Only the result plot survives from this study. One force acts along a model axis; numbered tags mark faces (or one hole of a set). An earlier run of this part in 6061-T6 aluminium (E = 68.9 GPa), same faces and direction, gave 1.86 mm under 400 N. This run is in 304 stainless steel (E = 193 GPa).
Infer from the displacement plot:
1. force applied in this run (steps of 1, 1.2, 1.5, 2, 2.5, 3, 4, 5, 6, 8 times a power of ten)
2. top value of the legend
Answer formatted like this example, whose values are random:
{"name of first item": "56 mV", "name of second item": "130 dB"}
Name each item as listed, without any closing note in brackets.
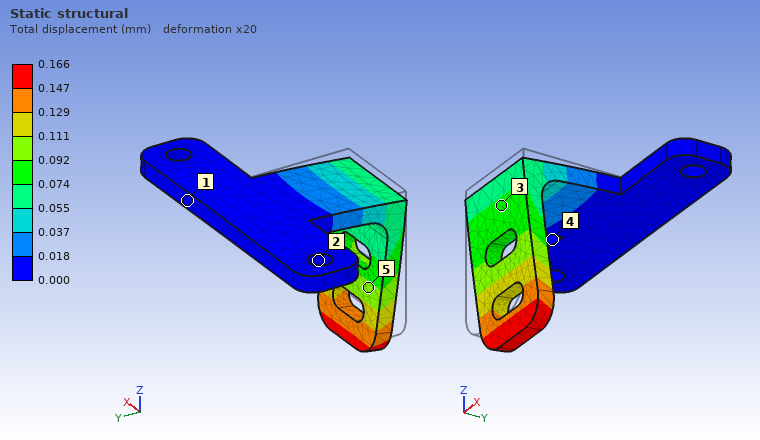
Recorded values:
{"force applied in this run": "100 N", "top value of the legend": "0.166 mm"}
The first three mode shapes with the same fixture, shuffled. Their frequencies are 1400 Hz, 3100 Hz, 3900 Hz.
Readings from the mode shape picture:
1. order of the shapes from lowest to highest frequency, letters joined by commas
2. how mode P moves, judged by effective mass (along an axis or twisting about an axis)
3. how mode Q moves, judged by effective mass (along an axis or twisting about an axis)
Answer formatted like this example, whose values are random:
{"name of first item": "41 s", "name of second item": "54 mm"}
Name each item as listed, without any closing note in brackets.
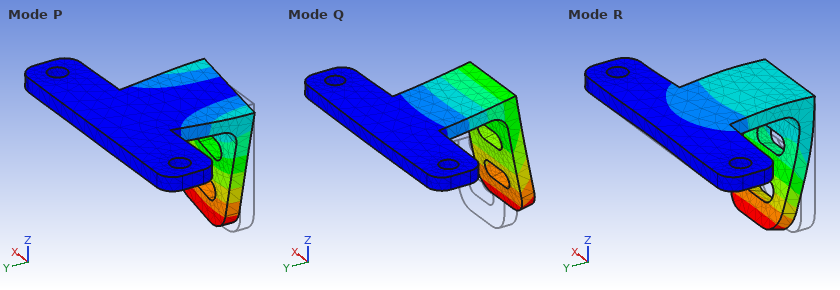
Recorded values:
{"order of the shapes from lowest to highest frequency, letters joined by commas": "Q, P, R", "how mode P moves, judged by effective mass": "along X", "how mode Q moves, judged by effective mass": "along Z"}
